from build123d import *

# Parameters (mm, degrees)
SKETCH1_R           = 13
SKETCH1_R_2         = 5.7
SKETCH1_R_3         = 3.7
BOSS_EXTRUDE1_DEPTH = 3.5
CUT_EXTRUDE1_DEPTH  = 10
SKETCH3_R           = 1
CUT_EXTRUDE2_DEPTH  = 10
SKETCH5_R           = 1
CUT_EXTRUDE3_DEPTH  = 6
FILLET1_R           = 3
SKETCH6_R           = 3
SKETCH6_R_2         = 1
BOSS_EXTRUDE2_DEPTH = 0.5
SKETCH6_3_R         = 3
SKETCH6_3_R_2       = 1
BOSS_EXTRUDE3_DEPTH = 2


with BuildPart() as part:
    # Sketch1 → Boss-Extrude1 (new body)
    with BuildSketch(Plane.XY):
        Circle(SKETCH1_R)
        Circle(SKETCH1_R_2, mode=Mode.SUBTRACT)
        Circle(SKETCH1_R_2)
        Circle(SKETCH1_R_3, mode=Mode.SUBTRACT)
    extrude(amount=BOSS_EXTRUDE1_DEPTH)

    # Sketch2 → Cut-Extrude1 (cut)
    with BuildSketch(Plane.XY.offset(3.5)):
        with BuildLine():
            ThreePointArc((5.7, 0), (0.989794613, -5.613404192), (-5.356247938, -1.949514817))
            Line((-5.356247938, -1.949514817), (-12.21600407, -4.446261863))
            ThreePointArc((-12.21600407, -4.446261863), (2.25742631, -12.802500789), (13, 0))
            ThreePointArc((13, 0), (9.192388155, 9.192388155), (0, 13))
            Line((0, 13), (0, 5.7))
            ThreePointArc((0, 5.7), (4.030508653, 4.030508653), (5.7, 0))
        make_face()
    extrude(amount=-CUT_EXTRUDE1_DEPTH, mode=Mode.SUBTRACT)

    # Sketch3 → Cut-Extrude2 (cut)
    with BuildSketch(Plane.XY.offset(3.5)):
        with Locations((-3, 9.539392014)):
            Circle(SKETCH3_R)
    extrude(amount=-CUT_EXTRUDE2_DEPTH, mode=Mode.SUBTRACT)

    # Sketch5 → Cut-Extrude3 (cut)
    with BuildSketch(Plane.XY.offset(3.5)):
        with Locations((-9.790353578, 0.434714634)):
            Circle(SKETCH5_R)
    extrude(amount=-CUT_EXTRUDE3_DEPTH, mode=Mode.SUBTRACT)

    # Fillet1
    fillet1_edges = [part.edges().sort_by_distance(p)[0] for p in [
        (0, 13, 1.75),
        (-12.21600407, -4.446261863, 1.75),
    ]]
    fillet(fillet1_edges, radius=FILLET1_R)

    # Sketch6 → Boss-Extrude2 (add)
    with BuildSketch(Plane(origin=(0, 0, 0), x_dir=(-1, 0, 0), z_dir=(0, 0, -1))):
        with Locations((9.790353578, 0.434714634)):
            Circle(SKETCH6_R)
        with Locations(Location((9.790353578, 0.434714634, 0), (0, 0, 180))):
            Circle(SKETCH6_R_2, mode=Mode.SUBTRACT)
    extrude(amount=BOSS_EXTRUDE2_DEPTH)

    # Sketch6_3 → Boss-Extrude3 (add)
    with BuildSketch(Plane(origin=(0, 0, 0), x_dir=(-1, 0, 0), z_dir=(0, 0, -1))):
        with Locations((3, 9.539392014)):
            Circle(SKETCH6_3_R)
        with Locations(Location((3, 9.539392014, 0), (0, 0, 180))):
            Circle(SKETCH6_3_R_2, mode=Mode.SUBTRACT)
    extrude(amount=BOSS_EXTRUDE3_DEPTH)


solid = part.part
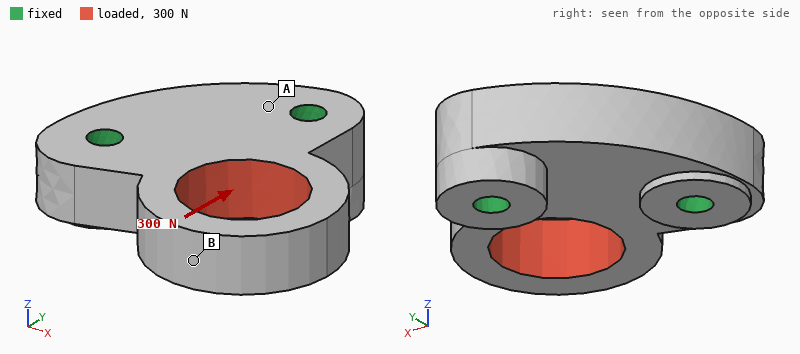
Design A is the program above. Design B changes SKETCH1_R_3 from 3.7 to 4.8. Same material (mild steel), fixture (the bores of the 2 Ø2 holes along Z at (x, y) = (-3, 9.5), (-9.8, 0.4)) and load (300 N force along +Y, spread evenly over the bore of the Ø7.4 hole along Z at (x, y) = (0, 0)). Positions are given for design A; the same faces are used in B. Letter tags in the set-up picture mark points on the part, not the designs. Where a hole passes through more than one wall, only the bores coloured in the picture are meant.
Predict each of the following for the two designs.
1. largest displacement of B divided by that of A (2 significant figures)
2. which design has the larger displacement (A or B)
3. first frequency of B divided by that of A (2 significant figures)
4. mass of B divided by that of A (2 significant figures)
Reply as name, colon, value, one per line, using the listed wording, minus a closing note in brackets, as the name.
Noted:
largest displacement of B divided by that of A: 8.9
which design has the larger displacement: B
first frequency of B divided by that of A: 0.68
mass of B divided by that of A: 0.85
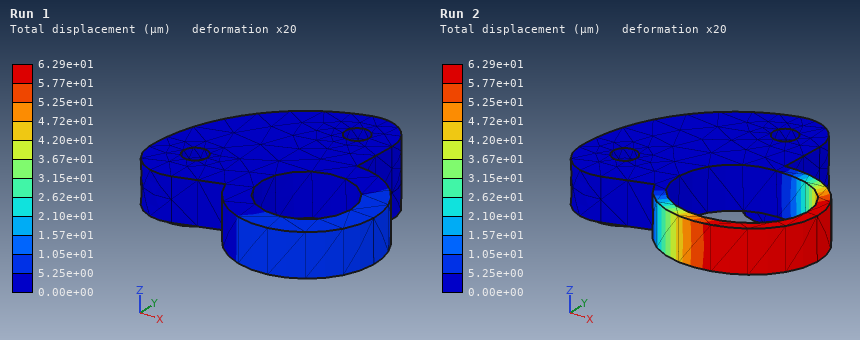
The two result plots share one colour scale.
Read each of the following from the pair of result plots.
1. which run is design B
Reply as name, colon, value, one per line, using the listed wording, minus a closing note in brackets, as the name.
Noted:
which run is design B: Run 2
